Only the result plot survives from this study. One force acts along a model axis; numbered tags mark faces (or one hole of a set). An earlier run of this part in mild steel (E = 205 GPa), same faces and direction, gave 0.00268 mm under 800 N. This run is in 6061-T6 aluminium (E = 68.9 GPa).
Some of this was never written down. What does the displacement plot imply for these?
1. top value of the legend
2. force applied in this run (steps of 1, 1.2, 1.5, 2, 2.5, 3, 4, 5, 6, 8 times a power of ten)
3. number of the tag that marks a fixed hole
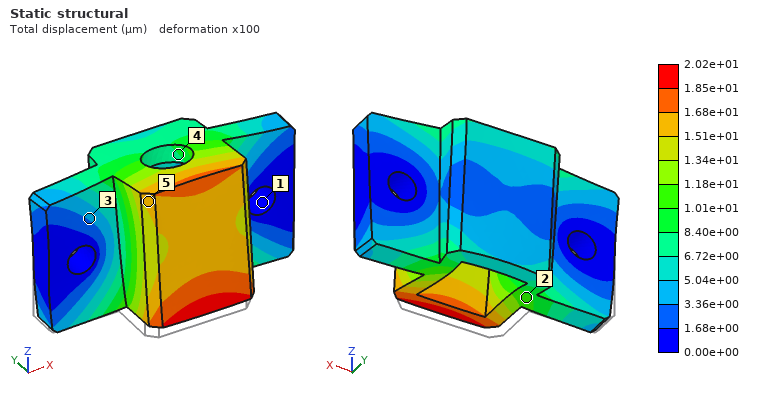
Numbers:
2.02e+01 µm
2 kN
1
